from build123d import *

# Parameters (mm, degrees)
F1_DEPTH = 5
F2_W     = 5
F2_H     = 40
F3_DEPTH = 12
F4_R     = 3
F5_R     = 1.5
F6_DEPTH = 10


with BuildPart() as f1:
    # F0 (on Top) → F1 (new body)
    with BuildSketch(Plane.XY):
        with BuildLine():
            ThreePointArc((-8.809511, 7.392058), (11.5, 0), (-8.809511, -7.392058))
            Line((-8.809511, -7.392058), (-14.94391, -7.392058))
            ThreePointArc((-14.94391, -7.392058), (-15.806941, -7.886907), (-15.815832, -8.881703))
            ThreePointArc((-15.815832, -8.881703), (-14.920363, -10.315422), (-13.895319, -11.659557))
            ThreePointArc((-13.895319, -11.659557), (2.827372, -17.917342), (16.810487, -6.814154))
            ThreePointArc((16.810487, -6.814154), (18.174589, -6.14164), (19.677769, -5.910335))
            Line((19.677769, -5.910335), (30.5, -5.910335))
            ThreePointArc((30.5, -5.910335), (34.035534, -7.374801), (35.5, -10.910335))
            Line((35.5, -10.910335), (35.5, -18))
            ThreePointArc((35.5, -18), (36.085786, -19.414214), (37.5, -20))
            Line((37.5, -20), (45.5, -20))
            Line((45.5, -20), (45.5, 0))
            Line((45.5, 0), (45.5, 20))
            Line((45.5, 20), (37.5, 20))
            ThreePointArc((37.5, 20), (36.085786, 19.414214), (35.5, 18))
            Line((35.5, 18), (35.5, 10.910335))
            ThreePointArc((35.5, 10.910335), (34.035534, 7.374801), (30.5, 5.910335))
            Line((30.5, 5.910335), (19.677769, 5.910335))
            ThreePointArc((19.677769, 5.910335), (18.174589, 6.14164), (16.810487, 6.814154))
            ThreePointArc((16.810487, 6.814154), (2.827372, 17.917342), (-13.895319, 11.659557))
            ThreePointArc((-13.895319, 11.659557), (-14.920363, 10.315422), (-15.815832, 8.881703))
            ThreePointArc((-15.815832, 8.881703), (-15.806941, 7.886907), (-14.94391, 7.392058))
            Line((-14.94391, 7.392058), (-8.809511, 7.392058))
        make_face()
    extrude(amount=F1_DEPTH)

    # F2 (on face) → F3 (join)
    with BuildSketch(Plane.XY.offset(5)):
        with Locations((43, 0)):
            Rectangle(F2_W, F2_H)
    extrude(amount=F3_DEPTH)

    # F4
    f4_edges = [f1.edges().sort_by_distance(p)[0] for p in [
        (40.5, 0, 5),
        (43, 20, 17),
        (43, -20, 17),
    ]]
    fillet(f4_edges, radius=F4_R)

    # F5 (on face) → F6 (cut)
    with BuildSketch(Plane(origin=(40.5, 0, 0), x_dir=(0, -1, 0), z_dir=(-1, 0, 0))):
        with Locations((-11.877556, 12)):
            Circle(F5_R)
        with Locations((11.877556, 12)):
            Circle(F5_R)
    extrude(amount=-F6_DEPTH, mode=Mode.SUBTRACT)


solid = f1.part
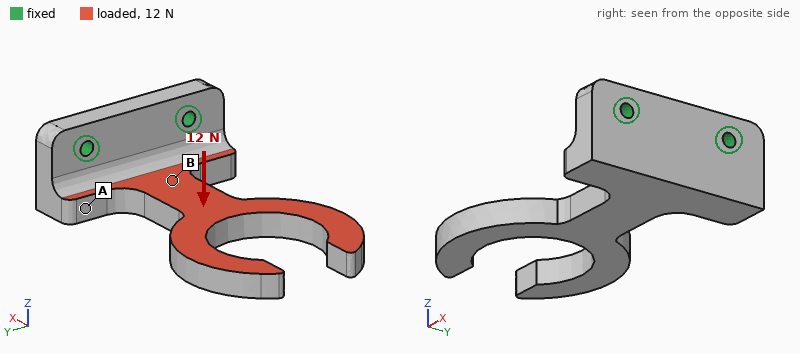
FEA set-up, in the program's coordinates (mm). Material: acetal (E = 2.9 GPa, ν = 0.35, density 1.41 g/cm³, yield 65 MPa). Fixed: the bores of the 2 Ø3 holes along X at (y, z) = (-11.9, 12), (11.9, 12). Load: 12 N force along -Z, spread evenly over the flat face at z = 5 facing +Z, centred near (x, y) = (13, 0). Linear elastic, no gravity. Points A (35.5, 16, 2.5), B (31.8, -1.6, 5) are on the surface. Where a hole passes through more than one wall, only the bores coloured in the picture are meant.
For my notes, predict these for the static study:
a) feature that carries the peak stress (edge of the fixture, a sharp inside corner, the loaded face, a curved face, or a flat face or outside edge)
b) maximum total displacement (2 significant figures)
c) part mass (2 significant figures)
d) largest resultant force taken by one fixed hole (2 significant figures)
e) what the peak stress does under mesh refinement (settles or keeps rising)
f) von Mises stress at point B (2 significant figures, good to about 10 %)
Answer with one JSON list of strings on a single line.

["edge of the fixture", "0.82 mm", "11 g", "7.5 N", "keeps rising", "4.4 MPa"]
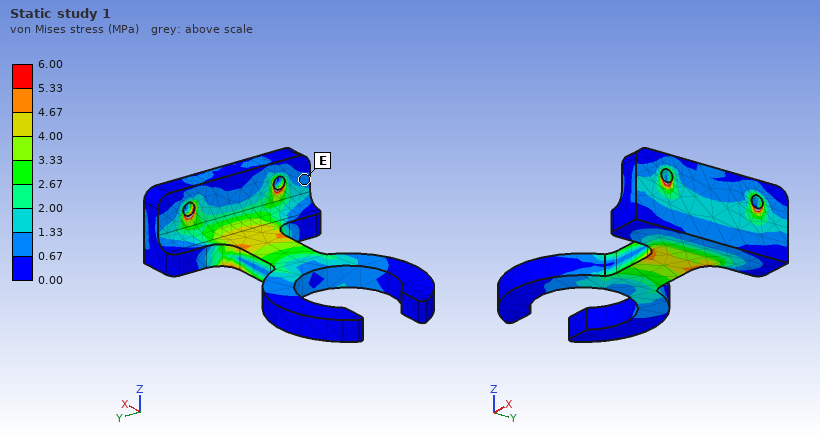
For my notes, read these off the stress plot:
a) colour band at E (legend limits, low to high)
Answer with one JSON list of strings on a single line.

["0.67 to 1.33 MPa"]
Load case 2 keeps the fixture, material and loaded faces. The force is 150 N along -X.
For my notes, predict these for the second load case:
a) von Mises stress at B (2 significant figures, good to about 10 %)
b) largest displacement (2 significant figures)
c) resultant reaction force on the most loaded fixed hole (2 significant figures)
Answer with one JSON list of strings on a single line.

["6.9 MPa", "0.76 mm", "75 N"]
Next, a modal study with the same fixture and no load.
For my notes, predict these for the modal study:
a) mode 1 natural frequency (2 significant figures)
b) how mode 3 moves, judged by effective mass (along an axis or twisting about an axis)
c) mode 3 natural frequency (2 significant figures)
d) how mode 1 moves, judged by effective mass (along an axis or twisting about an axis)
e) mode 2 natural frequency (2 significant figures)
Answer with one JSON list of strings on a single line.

["320 Hz", "along Y", "690 Hz", "along Z", "660 Hz"]
